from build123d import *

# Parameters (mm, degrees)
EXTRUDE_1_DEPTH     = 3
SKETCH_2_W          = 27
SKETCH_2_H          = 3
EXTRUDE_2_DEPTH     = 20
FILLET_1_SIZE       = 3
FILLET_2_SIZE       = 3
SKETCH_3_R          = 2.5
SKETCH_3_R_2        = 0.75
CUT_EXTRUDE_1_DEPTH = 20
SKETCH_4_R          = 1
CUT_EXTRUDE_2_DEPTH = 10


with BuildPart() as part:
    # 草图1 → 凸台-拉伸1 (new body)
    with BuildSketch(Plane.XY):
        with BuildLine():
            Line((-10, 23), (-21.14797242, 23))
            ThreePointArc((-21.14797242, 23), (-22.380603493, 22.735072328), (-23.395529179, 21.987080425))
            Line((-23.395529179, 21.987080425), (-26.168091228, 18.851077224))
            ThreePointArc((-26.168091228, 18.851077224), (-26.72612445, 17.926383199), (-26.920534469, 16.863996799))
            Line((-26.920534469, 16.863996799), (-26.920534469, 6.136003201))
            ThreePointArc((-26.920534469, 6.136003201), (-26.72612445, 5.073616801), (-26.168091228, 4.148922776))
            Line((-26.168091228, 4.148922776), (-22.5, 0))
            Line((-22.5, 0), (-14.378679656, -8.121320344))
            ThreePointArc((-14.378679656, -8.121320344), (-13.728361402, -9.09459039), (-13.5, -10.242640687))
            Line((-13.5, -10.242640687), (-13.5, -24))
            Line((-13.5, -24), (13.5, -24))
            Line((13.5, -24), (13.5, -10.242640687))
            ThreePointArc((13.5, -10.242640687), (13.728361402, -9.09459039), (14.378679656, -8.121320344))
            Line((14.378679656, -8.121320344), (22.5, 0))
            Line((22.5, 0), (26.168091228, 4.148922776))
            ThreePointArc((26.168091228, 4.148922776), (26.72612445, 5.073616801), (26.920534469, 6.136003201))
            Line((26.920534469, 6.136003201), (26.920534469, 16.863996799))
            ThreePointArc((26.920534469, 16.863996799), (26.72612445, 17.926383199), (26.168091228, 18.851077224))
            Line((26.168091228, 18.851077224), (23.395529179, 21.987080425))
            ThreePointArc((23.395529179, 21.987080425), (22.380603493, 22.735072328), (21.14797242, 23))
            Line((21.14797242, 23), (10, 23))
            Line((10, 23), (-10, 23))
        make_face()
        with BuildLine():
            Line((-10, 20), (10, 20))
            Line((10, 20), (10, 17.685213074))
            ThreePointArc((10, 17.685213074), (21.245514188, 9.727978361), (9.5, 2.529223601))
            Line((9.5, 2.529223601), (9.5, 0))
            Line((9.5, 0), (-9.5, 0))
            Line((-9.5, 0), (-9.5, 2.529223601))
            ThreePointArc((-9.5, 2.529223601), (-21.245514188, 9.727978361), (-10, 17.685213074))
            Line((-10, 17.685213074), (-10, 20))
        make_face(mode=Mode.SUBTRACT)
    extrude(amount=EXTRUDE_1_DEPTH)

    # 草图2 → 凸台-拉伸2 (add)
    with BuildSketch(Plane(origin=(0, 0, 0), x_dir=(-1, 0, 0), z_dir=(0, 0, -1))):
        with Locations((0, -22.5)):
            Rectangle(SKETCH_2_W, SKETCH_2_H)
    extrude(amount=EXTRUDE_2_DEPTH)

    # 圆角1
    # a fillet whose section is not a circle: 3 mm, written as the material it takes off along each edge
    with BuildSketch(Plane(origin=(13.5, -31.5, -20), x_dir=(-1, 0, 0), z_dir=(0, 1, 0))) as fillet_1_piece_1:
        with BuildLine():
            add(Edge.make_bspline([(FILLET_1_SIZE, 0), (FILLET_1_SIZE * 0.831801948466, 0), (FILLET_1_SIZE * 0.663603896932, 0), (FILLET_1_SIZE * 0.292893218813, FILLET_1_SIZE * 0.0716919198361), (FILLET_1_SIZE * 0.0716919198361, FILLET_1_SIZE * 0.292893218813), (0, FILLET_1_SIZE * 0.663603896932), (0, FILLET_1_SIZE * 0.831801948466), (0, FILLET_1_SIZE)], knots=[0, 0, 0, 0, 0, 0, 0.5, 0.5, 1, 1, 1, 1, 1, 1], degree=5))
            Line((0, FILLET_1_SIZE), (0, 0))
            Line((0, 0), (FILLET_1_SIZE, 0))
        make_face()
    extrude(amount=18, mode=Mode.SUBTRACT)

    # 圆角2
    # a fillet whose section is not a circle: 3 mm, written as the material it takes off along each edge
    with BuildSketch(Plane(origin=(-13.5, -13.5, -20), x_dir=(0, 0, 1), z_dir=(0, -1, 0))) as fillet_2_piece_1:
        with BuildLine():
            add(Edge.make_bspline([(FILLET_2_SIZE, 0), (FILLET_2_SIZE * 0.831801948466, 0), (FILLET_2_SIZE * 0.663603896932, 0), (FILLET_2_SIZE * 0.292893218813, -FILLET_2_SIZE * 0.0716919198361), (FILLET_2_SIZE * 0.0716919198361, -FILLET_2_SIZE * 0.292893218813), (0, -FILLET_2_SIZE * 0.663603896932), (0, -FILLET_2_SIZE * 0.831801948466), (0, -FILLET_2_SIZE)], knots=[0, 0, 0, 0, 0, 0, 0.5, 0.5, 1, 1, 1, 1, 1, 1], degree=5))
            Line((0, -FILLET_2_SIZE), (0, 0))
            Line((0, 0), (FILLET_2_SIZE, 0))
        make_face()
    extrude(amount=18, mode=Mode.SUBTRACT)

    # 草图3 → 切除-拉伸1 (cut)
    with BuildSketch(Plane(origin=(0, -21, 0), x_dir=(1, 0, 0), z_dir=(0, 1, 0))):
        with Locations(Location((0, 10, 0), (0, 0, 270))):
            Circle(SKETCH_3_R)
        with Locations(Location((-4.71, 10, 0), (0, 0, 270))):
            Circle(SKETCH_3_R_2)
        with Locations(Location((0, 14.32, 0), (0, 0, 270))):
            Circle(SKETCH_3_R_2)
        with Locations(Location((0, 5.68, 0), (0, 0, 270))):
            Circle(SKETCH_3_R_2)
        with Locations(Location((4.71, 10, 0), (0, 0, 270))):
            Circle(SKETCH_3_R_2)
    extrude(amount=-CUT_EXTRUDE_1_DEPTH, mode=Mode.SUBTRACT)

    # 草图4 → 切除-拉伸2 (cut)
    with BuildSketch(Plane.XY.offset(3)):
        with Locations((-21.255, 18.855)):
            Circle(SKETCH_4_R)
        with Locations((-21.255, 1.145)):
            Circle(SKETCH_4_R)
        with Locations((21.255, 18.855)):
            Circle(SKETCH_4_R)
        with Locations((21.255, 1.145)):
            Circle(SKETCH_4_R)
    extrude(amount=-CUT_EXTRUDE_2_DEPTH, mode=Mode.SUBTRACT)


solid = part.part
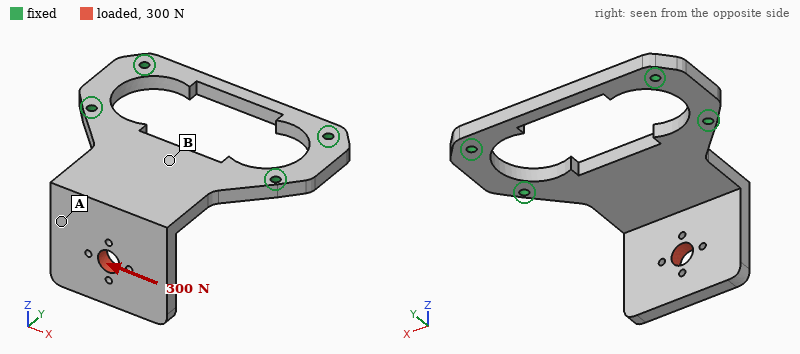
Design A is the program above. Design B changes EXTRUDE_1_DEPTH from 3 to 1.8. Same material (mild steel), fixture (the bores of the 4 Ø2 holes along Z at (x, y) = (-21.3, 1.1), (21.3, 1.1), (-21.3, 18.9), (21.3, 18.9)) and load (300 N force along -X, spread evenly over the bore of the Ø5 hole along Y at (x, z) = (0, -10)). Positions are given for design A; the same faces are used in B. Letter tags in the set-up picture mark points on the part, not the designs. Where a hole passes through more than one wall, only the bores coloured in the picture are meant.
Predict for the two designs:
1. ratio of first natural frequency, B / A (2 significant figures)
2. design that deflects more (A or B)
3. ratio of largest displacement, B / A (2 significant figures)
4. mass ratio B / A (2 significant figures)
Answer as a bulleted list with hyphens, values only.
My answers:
- 0.52
- B
- 3.4
- 0.72
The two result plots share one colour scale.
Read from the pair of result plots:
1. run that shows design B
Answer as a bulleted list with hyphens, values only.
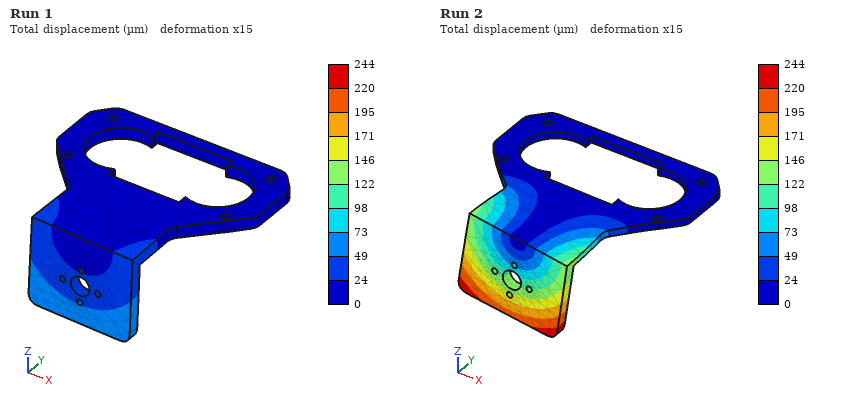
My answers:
- Run 2
